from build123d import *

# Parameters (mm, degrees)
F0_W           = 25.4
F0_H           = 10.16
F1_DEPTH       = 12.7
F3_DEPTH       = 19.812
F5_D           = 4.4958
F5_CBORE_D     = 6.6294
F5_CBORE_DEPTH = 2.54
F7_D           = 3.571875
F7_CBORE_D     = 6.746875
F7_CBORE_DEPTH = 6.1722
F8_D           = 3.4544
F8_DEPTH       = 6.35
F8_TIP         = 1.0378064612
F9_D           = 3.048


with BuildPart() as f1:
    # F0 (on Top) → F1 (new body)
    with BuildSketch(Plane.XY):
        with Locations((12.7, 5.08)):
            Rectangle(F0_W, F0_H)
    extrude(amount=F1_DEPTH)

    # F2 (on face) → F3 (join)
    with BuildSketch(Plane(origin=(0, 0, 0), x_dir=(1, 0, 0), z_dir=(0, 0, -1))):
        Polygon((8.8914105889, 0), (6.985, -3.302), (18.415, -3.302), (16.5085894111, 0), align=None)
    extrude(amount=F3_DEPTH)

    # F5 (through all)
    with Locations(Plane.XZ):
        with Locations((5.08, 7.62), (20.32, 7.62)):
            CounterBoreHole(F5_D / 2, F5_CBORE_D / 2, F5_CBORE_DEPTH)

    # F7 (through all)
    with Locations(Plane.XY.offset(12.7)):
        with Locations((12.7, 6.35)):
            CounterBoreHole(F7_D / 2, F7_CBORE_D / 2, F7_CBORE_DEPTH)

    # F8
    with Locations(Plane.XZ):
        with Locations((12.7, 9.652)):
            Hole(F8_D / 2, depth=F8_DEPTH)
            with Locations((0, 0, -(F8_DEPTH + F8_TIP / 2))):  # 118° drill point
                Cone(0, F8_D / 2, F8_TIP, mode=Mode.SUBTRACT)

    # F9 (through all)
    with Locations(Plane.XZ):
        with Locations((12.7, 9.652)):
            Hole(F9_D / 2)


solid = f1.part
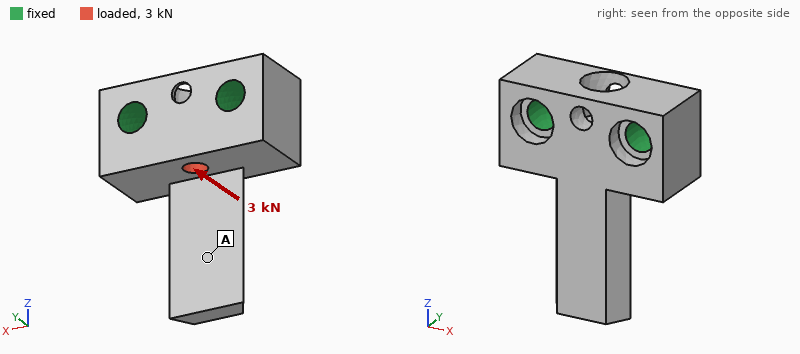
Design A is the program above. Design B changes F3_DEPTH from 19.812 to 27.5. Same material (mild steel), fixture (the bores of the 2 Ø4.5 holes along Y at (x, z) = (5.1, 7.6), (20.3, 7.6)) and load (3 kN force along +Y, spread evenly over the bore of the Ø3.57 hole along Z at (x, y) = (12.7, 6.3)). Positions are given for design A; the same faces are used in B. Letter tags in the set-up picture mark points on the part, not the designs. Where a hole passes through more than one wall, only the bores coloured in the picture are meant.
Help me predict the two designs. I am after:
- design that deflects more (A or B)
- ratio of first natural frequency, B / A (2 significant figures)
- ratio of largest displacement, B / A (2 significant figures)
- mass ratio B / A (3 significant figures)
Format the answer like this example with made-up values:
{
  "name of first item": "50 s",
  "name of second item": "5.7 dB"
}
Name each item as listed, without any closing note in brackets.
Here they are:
{
  "design that deflects more": "B",
  "ratio of first natural frequency, B / A": "0.55",
  "ratio of largest displacement, B / A": "1.3",
  "mass ratio B / A": "1.08"
}
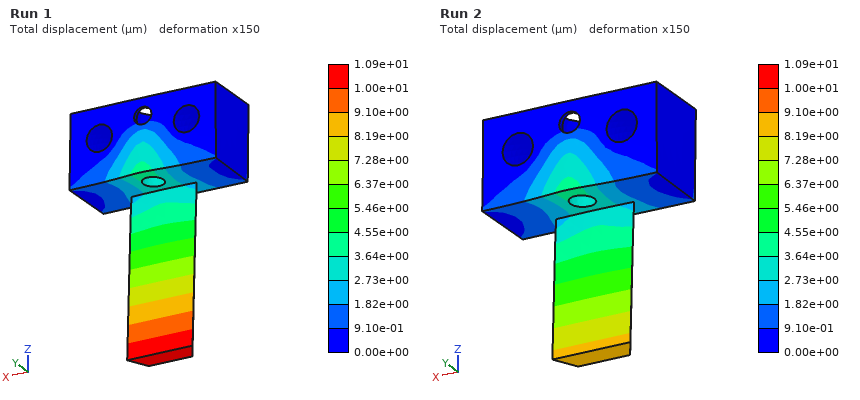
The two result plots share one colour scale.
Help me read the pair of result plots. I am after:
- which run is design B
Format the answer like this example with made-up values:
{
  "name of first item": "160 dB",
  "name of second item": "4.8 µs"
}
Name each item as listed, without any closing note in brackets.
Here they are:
{
  "which run is design B": "Run 1"
}
